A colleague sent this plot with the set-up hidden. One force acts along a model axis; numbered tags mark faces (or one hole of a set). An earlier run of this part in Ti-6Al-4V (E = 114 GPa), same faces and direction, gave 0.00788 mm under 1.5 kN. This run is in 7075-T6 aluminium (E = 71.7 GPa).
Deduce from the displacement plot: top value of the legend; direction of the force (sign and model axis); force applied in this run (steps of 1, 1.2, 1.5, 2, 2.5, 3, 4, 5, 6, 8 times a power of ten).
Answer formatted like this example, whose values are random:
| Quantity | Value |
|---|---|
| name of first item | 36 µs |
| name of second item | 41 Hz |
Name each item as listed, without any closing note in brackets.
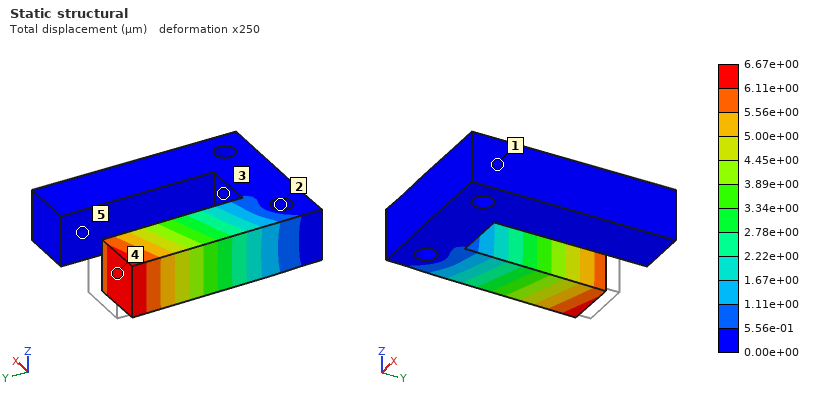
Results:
| Quantity | Value |
|---|---|
| top value of the legend | 6.67e+00 µm |
| direction of the force | -Y |
| force applied in this run | 800 N |
